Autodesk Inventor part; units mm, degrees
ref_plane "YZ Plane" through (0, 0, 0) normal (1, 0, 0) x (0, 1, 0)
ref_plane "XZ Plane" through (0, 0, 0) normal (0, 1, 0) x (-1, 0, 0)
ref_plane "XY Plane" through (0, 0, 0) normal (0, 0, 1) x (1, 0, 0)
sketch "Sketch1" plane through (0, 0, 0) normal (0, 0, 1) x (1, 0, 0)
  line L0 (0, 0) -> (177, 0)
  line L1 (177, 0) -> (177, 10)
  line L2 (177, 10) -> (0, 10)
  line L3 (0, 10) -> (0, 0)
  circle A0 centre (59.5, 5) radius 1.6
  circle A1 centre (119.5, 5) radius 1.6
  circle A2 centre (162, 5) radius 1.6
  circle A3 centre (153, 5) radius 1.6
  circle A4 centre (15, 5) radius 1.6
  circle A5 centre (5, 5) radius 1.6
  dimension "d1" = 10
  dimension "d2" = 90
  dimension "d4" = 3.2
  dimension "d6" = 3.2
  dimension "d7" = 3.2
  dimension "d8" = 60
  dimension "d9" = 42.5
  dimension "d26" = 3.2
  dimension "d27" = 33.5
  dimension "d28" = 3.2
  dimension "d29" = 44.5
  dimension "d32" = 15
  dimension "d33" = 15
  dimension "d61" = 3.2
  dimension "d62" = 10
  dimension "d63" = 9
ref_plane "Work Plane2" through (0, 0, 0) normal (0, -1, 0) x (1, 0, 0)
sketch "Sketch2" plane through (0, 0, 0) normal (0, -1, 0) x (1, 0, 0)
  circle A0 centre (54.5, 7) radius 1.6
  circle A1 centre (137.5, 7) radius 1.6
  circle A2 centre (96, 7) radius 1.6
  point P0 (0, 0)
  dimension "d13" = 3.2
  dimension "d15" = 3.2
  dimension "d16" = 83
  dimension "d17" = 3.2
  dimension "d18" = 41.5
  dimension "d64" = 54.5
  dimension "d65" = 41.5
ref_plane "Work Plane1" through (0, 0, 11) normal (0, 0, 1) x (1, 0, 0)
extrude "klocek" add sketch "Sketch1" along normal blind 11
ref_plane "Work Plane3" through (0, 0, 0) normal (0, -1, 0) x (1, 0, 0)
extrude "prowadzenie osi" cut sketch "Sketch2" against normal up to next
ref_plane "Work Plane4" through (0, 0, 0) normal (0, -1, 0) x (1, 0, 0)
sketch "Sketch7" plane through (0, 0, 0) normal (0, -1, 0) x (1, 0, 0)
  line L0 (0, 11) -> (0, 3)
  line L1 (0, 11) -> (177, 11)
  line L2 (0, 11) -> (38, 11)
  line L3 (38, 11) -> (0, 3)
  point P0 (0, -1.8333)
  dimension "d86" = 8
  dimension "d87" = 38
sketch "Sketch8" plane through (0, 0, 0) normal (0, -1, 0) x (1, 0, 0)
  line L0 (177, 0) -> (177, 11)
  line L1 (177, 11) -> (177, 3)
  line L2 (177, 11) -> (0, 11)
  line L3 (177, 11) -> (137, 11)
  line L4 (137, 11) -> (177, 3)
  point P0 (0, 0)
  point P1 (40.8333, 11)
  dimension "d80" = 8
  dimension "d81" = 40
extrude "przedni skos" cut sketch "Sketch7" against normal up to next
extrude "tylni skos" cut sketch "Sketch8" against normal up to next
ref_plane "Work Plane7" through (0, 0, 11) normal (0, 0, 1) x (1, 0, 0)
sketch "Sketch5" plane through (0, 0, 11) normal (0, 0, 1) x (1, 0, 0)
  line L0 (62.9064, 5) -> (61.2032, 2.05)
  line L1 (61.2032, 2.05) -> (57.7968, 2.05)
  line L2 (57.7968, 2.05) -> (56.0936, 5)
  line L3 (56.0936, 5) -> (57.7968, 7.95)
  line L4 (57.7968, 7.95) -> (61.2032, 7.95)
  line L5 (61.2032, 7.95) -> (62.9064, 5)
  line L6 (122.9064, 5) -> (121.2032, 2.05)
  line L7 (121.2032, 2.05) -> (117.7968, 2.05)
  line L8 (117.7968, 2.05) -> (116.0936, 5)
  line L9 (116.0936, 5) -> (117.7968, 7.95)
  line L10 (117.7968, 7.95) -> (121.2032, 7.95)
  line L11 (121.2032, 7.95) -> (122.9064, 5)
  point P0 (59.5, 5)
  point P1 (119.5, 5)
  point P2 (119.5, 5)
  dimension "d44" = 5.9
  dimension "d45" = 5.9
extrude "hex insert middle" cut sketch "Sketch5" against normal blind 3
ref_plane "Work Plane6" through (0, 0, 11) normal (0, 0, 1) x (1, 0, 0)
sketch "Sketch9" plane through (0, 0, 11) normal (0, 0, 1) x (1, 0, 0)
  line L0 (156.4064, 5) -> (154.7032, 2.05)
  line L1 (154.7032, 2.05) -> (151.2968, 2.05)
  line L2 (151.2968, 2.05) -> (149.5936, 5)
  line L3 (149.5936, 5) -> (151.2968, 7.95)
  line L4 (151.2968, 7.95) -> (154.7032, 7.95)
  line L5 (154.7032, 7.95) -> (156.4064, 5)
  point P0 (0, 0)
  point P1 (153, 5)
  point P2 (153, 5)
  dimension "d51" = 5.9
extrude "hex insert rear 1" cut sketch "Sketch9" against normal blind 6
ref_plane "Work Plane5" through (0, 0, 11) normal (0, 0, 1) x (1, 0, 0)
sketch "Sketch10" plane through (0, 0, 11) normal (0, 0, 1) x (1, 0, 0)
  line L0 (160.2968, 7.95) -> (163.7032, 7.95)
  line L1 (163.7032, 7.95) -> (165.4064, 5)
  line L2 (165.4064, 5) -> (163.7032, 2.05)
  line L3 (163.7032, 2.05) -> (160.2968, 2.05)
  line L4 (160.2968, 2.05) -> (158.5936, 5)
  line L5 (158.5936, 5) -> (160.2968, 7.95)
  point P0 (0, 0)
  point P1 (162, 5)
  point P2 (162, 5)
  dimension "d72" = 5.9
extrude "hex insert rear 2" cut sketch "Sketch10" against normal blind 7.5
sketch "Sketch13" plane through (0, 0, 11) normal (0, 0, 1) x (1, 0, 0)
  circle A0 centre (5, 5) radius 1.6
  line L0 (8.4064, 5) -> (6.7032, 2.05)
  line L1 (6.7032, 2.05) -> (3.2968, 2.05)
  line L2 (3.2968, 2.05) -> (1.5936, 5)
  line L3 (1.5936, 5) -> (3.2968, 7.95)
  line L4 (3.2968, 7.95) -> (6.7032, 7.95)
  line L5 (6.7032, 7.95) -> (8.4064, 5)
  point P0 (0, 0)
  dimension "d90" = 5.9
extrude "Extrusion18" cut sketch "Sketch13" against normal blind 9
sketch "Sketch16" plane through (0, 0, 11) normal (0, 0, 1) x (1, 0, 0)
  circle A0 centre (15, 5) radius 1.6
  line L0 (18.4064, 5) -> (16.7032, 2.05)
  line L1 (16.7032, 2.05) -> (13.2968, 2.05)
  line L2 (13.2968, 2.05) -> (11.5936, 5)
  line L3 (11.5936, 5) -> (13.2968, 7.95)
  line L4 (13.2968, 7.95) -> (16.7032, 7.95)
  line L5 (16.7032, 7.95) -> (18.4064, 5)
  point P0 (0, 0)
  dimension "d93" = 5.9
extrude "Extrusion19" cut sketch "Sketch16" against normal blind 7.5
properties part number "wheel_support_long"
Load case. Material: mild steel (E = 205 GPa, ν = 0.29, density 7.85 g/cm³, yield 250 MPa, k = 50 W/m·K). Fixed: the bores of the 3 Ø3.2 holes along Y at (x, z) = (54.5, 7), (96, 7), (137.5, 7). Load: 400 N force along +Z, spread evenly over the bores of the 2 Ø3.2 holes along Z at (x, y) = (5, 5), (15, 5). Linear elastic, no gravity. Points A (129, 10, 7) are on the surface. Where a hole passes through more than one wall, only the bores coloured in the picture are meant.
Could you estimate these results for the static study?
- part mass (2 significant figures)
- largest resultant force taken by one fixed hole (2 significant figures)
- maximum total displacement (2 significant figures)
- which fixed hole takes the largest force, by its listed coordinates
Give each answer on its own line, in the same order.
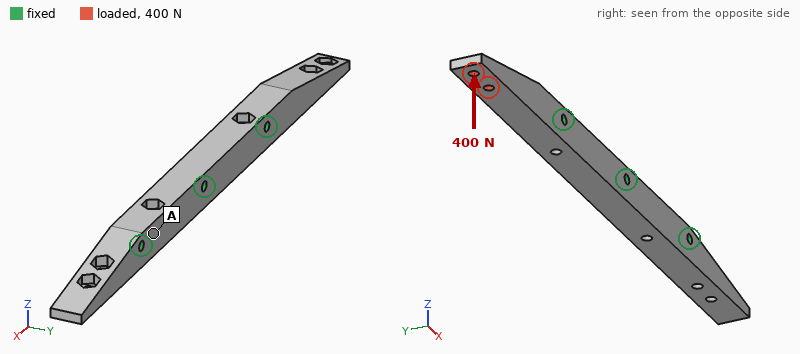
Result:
120 g
710 N
0.11 mm
(54.5, 7)
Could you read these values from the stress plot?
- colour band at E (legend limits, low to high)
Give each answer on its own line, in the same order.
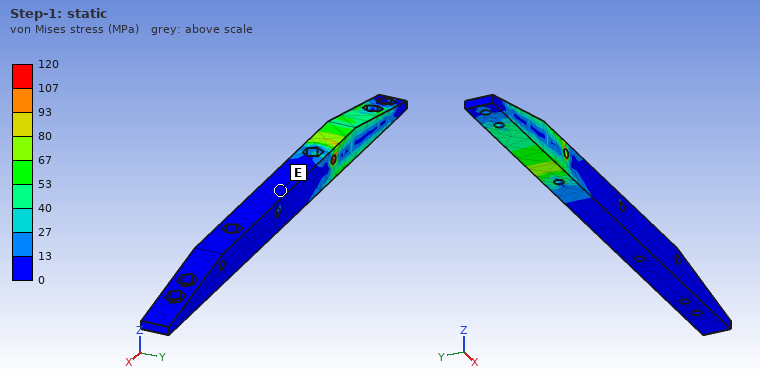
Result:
0 to 13 MPa
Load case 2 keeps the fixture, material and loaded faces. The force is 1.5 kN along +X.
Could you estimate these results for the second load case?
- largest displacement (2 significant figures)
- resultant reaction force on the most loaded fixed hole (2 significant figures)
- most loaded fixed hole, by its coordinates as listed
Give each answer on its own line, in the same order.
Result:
61 µm
1.3 kN
(54.5, 7)
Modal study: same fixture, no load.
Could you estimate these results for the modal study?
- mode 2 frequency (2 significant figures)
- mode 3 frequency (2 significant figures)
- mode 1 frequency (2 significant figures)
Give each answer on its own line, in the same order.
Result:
4000 Hz
5400 Hz
3800 Hz
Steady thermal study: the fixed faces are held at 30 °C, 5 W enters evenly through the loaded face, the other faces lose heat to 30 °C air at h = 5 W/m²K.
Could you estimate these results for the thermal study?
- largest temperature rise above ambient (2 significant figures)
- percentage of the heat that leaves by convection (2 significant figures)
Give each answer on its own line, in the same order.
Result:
57 K
5.4 %
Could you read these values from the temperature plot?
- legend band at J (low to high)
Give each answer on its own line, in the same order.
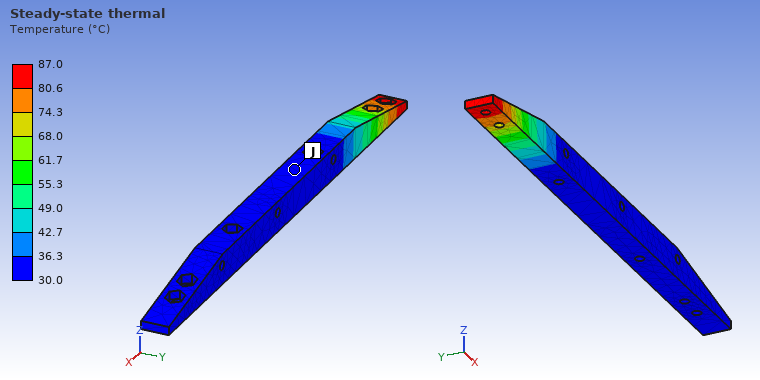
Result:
30.0 to 36.3 °C
